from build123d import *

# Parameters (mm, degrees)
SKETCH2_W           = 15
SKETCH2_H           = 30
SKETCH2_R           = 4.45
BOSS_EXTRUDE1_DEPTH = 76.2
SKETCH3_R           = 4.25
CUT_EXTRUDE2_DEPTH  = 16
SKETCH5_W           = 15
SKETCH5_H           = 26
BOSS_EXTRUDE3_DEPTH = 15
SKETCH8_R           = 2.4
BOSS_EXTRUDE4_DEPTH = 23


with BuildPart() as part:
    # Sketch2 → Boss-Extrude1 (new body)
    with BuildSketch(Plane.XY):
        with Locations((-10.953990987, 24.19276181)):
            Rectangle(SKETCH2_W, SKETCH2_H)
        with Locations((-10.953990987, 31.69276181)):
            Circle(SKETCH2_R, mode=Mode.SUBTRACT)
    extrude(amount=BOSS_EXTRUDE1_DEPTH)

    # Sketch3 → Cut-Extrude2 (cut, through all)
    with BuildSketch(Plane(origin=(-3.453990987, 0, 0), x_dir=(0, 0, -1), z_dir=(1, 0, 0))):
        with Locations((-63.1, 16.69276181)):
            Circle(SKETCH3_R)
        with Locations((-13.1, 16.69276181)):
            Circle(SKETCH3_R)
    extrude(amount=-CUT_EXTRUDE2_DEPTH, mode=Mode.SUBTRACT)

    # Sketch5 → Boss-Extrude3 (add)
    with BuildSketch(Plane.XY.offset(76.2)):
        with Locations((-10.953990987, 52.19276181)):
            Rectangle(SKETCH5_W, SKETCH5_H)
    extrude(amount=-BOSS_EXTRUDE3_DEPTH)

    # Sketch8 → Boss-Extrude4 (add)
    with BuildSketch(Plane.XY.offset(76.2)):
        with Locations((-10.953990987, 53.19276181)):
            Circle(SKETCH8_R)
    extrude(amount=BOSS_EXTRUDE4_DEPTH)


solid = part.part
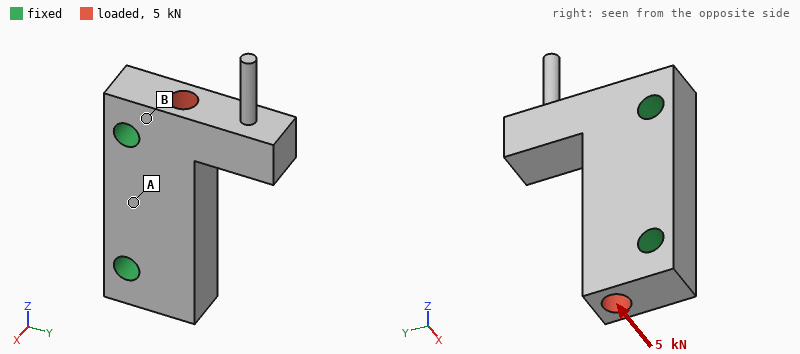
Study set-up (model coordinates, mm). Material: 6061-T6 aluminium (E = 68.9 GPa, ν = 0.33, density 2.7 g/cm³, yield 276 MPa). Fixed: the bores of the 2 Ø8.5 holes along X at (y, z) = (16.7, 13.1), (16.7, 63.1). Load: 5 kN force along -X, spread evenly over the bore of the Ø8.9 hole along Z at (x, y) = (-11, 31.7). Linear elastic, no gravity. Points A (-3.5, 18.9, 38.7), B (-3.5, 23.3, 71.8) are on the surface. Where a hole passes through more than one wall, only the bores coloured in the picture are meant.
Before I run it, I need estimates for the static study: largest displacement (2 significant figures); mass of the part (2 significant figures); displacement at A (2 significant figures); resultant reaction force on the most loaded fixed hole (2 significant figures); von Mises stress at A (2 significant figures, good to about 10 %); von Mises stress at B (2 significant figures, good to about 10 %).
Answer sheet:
32 µm
92 g
6.7 µm
2.5 kN
8.1 MPa
17 MPa
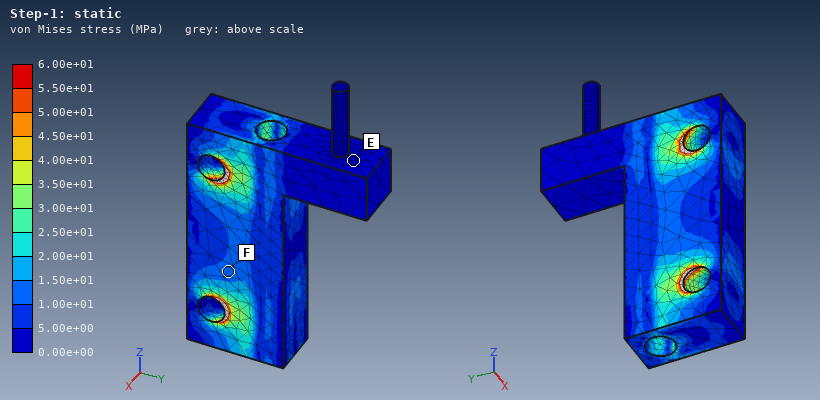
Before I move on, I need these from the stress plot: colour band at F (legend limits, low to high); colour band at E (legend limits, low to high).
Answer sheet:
1.00e+01 to 1.50e+01 MPa
0.00e+00 to 5.00e+00 MPa
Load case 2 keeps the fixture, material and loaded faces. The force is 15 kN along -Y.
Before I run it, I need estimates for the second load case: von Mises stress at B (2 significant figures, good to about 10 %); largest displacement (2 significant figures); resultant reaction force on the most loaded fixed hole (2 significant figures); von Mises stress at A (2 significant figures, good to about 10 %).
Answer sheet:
14 MPa
14 µm
7.6 kN
4.6 MPa
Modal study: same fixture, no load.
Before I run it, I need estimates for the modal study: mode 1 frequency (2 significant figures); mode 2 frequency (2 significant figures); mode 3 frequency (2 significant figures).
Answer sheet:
5000 Hz
5400 Hz
6200 Hz
